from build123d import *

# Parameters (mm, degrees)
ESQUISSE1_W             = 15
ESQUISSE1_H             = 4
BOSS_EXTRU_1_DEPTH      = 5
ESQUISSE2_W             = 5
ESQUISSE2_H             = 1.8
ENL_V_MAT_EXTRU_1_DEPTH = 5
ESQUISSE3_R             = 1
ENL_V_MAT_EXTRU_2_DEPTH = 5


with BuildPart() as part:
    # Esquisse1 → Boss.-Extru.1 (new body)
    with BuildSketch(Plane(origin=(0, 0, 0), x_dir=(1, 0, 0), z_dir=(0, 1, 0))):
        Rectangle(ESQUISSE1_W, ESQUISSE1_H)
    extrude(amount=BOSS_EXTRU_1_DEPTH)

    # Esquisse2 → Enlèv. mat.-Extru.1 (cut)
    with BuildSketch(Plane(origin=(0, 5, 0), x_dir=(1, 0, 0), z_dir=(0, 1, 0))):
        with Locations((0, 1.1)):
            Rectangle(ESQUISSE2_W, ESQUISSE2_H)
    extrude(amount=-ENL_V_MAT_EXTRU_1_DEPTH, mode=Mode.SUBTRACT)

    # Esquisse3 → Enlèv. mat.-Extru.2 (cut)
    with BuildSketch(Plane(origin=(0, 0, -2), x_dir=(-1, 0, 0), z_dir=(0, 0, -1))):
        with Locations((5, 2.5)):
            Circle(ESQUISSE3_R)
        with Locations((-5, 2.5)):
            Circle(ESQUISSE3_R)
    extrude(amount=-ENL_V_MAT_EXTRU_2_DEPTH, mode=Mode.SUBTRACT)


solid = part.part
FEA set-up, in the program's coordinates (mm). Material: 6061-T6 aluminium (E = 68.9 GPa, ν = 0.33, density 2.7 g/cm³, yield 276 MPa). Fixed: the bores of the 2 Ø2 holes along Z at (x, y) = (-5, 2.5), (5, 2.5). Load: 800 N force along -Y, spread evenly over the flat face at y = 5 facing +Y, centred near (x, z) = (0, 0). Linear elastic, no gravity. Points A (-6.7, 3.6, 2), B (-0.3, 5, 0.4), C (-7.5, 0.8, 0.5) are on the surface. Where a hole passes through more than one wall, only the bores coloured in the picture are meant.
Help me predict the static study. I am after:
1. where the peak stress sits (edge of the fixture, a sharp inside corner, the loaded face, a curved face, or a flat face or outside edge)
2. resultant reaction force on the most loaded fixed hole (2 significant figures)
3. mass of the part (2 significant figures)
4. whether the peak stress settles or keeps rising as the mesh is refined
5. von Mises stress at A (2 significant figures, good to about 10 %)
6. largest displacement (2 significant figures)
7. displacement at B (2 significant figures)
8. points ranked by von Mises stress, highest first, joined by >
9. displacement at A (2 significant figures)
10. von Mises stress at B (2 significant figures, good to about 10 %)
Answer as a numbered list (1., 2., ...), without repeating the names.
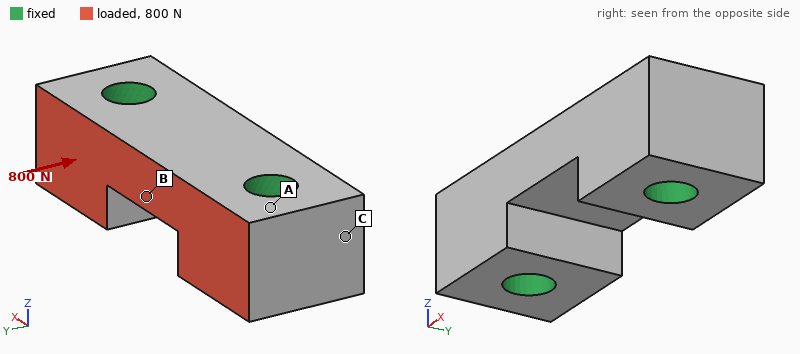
1. edge of the fixture
2. 400 N
3. 0.62 g
4. keeps rising
5. 12 MPa
6. 2.3 µm
7. 2.0 µm
8. B > A > C
9. 0.38 µm
10. 22 MPa
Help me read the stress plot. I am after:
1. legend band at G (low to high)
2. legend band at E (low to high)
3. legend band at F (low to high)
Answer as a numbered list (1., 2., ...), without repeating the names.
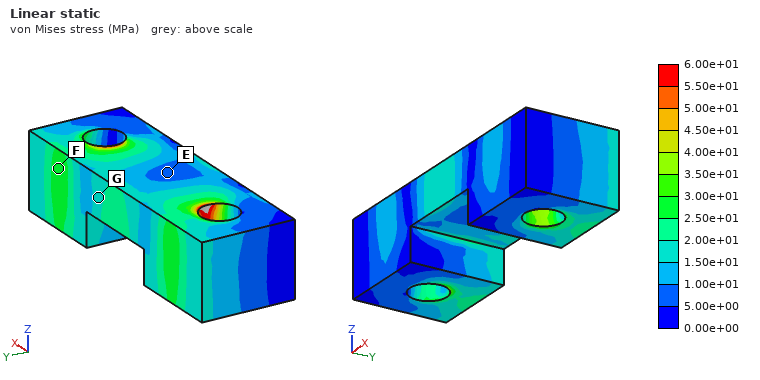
1. 1.50e+01 to 2.00e+01 MPa
2. 5.00e+00 to 1.00e+01 MPa
3. 2.50e+01 to 3.00e+01 MPa
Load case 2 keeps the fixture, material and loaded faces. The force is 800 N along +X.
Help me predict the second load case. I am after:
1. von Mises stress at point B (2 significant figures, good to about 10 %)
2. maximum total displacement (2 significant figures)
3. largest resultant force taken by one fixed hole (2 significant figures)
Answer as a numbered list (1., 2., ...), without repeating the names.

1. 27 MPa
2. 3.0 µm
3. 410 N
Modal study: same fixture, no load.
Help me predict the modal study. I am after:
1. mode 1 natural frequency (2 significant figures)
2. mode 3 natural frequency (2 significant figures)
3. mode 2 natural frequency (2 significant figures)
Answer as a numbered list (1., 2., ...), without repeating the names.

1. 140 kHz
2. 170 kHz
3. 140 kHz
